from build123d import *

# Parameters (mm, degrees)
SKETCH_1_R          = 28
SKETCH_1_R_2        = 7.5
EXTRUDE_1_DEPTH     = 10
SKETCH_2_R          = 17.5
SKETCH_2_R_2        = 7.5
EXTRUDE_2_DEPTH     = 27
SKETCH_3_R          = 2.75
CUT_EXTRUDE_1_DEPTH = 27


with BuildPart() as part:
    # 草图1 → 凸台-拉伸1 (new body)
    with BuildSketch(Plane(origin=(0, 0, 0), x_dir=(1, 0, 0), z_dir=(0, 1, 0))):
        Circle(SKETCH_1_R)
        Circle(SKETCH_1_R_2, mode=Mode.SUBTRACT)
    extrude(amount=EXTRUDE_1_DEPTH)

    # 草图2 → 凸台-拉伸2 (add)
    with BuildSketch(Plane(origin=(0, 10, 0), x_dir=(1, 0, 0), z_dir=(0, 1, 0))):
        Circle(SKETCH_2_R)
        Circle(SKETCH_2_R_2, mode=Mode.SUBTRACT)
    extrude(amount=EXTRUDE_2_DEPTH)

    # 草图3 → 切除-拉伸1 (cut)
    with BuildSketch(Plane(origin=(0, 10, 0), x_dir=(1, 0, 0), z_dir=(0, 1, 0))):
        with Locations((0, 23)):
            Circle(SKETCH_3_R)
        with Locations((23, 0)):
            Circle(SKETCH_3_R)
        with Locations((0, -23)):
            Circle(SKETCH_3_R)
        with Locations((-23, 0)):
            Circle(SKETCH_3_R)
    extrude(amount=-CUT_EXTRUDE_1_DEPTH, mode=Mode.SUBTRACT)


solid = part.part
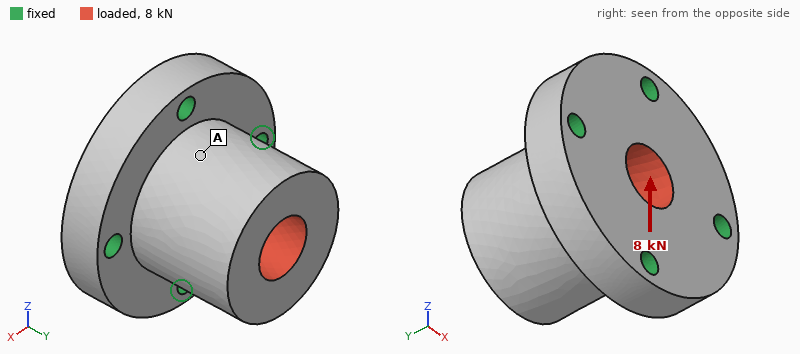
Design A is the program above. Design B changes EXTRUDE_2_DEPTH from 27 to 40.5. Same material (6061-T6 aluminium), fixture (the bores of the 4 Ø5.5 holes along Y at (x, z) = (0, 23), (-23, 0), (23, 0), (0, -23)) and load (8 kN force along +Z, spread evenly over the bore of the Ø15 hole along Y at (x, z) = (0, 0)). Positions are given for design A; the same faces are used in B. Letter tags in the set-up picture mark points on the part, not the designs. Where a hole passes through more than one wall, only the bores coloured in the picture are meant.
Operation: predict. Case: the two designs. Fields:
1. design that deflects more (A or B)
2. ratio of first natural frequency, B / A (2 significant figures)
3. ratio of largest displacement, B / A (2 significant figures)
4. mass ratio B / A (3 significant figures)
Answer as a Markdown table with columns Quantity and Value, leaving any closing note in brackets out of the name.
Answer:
| Quantity | Value |
|---|---|
| design that deflects more | B |
| ratio of first natural frequency, B / A | 0.60 |
| ratio of largest displacement, B / A | 2.1 |
| mass ratio B / A | 1.25 |
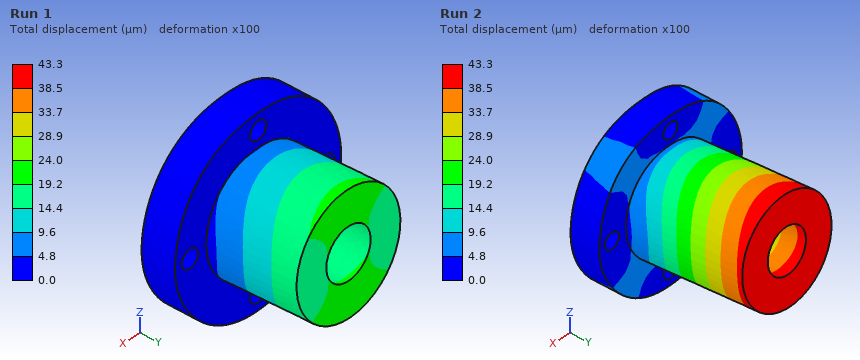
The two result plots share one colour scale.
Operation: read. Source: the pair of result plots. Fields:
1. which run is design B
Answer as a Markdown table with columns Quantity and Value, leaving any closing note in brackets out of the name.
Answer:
| Quantity | Value |
|---|---|
| which run is design B | Run 2 |
